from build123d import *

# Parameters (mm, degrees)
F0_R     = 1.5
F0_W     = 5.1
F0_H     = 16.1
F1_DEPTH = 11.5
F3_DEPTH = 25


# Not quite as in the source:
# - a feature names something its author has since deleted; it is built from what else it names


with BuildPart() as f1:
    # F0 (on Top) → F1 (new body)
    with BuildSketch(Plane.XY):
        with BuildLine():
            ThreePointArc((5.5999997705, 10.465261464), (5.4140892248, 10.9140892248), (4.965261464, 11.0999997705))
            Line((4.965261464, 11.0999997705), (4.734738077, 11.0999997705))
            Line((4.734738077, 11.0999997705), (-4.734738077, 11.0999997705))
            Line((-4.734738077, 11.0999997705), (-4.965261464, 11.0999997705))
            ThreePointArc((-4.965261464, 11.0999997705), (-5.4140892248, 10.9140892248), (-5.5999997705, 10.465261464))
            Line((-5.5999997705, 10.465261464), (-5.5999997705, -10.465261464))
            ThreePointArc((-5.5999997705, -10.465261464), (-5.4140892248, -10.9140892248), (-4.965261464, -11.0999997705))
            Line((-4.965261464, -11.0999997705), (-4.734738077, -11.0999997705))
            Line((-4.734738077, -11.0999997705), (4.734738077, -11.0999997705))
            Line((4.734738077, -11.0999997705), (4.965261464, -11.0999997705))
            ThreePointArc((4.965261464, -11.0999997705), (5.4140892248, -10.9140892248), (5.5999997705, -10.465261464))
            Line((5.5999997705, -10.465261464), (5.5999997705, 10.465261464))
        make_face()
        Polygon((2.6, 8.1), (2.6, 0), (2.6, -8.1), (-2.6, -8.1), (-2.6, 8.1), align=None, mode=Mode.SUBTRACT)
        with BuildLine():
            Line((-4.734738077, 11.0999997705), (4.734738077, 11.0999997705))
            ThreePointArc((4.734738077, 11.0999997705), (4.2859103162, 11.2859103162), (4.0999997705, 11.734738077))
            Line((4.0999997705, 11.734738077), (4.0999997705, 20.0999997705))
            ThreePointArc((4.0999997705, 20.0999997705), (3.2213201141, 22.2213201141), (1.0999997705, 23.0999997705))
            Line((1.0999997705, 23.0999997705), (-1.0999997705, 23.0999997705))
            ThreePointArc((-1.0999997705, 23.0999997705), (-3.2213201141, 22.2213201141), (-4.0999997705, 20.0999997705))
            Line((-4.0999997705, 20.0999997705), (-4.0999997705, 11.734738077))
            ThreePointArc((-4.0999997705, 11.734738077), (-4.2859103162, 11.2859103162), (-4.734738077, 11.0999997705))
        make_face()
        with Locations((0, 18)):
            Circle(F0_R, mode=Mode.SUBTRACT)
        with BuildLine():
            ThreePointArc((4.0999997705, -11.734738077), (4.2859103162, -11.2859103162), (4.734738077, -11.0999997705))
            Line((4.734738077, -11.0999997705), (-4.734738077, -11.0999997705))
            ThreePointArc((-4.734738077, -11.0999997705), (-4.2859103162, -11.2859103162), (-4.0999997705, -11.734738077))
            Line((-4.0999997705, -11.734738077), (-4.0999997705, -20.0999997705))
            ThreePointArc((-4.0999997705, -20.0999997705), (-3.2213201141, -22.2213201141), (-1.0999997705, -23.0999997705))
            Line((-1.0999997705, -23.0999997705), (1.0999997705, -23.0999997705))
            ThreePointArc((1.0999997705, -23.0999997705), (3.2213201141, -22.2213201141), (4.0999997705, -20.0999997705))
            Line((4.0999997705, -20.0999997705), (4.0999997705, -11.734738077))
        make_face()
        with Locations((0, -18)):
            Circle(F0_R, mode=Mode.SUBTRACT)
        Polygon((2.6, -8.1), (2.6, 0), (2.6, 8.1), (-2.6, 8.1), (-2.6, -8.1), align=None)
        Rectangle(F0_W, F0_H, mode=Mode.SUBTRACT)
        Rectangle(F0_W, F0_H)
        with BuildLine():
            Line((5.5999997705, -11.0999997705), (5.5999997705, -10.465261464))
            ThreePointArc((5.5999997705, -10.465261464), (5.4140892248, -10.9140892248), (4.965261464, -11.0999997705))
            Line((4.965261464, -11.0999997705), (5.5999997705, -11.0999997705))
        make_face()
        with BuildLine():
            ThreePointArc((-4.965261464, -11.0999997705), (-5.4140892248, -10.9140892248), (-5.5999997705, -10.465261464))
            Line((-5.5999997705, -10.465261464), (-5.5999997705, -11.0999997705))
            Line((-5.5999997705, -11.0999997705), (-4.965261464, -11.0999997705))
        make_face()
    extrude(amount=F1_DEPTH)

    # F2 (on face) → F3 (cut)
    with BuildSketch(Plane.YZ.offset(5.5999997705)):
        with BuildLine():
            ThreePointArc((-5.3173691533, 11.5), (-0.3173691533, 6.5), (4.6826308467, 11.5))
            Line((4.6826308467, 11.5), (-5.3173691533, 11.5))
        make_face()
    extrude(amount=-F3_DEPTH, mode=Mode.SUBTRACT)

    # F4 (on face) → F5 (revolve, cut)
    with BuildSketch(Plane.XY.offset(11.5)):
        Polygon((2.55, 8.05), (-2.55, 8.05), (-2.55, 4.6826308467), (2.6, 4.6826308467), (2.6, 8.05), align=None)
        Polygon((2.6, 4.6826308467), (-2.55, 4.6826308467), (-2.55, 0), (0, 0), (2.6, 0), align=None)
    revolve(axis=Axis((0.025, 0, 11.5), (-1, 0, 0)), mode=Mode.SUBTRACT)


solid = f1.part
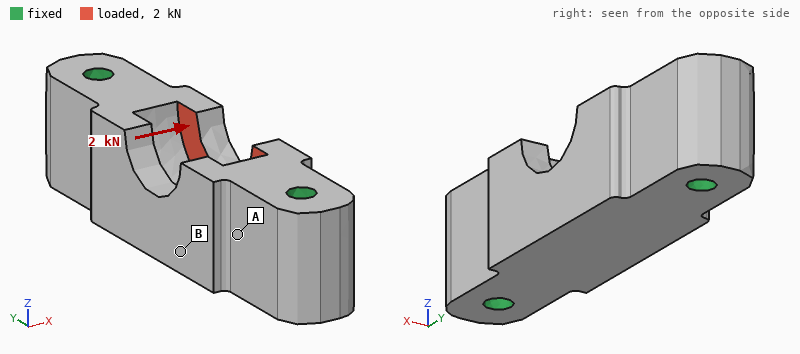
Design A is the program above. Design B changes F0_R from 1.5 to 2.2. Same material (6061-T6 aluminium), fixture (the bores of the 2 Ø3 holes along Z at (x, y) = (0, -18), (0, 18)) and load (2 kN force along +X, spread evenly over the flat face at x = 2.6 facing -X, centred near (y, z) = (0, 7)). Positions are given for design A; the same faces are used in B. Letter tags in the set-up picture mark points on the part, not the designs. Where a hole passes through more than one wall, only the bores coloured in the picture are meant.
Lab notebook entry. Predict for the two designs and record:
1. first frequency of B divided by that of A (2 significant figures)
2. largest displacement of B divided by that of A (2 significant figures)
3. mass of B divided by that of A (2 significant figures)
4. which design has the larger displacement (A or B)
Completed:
1.1
0.89
0.95
A
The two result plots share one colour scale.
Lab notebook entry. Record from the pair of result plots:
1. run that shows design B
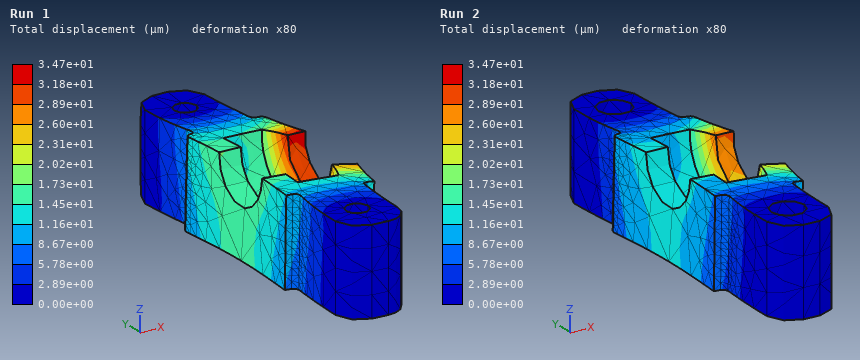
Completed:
Run 2
